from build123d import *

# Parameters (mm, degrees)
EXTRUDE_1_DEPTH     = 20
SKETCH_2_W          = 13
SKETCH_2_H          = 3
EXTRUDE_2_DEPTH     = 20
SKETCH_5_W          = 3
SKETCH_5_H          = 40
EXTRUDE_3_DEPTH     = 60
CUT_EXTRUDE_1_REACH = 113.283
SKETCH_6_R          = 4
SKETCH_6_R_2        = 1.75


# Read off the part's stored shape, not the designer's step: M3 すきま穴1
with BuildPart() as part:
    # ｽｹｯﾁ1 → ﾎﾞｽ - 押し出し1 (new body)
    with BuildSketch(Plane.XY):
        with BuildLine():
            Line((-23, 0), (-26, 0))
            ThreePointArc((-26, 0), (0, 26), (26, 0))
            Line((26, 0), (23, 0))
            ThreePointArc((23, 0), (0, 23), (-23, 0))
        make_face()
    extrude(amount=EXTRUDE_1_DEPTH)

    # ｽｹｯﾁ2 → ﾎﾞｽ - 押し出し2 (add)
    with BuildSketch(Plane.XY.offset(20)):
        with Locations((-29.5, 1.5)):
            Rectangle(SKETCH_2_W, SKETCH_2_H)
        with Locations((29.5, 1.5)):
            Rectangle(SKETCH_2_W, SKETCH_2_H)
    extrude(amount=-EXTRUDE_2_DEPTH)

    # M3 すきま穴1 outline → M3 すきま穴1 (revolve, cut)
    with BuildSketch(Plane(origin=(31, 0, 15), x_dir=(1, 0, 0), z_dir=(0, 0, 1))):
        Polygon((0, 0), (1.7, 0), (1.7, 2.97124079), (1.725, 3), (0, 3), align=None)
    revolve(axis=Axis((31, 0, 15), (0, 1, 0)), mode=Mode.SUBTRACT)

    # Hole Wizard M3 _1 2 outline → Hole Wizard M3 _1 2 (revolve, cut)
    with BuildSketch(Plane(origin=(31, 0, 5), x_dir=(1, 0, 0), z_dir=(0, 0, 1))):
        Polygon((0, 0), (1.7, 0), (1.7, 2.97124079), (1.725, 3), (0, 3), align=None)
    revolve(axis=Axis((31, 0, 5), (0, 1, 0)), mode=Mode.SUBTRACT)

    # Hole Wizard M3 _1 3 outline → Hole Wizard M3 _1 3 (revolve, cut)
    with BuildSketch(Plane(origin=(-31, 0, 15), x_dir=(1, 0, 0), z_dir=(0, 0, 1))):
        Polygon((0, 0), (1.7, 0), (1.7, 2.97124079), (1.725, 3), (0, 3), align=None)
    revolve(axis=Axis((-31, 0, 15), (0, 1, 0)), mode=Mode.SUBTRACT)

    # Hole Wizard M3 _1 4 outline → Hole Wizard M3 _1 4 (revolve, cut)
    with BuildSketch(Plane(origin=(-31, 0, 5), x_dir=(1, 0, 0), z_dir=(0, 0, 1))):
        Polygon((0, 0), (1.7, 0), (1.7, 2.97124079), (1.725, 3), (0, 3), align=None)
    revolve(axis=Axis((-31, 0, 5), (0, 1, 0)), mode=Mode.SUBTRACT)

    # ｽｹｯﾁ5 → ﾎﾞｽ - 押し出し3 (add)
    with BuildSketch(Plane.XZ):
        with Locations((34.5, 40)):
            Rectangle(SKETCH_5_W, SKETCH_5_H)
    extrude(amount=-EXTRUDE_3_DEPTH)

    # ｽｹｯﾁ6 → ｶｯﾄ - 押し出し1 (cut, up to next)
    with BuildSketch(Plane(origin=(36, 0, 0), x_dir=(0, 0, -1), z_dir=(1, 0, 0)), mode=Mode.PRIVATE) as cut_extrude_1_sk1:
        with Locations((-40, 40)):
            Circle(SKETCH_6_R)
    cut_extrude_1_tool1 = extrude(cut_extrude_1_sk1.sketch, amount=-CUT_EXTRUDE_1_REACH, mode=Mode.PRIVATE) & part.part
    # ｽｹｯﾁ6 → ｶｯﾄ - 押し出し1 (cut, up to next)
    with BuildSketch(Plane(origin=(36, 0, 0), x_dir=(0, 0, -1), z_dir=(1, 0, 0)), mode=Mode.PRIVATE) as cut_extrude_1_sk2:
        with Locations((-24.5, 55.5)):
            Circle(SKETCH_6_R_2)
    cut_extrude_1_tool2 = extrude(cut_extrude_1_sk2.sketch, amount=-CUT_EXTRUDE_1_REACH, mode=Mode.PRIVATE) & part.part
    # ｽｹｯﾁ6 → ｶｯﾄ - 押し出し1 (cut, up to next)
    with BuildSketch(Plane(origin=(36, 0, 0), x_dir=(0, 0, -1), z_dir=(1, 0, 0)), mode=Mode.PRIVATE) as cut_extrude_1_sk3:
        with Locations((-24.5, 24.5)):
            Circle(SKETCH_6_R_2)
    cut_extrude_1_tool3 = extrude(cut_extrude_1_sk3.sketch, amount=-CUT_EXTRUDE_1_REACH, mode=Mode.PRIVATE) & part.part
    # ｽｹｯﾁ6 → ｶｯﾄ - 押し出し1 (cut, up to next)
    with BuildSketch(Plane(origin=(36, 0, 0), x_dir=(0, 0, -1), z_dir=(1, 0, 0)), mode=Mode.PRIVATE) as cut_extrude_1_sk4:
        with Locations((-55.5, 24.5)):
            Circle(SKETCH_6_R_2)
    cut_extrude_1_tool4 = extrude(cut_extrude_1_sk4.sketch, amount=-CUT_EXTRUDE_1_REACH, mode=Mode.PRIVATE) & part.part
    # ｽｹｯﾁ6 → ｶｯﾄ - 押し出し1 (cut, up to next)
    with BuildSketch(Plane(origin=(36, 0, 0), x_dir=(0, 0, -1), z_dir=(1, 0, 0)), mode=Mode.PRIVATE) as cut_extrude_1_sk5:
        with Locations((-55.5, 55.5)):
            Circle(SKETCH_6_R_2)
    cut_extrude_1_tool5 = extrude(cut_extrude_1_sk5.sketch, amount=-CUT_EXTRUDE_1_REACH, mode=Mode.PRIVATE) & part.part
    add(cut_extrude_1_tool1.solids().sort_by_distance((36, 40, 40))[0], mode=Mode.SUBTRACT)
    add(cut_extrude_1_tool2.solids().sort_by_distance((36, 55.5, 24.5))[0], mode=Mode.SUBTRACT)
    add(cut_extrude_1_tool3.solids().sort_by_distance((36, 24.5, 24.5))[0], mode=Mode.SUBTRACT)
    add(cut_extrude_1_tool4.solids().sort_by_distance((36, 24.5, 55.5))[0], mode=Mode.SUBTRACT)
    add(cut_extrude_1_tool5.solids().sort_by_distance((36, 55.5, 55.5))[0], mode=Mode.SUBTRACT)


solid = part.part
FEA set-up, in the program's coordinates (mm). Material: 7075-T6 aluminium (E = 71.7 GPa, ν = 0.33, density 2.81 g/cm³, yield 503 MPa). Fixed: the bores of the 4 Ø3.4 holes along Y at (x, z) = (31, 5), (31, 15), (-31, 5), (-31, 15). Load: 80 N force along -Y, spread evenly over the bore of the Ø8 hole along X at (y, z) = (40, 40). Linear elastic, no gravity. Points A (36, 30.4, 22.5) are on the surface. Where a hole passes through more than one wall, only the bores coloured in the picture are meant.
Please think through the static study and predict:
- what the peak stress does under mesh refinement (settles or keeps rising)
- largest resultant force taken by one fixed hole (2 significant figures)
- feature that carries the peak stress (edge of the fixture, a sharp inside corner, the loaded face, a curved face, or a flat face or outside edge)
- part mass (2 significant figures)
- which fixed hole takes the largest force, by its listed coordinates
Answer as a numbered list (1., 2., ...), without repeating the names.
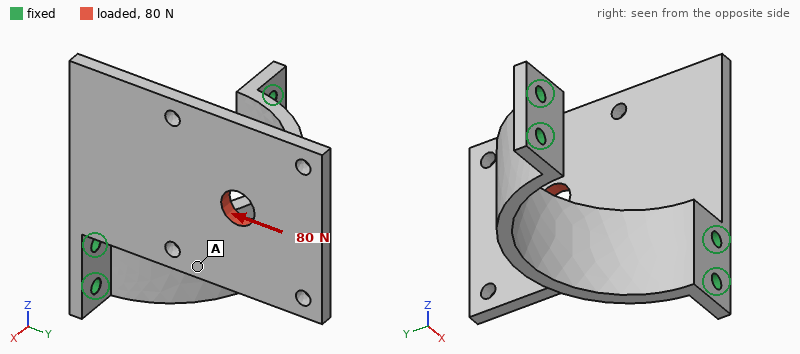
1. keeps rising
2. 110 N
3. a sharp inside corner
4. 36 g
5. (31, 15)
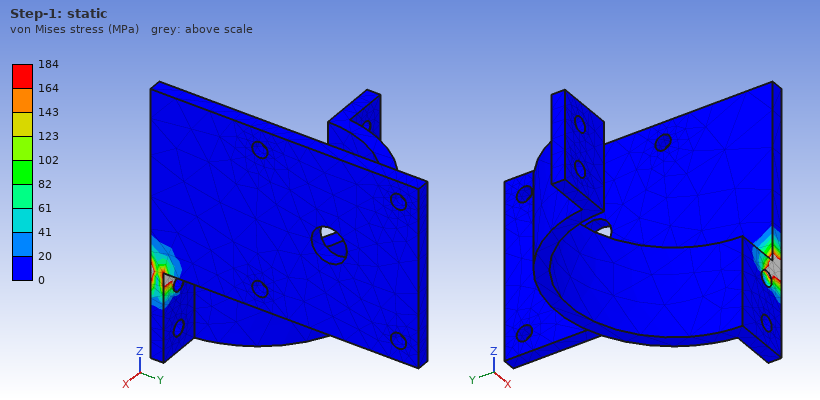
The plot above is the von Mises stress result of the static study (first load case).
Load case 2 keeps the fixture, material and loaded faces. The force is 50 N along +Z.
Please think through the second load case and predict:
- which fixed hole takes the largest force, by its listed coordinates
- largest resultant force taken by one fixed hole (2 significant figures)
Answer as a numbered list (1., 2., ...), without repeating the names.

1. (31, 15)
2. 52 N
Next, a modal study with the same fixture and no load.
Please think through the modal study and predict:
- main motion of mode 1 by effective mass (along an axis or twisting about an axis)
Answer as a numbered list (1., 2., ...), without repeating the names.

1. along X
